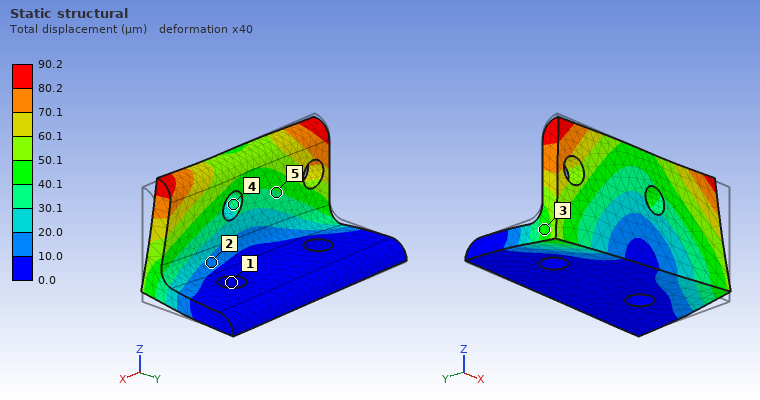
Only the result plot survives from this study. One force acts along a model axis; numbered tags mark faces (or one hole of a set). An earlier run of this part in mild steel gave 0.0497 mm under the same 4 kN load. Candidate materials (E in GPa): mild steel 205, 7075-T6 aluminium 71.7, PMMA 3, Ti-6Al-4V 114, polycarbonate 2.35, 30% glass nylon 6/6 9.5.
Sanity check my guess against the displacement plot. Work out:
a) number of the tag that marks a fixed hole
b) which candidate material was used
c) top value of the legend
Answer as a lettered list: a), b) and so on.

a) 1
b) Ti-6Al-4V
c) 90.2 µm
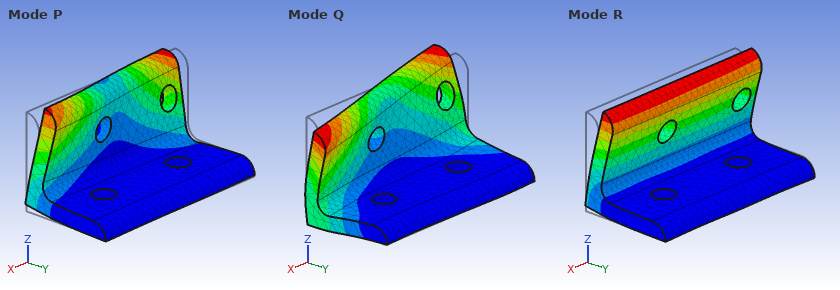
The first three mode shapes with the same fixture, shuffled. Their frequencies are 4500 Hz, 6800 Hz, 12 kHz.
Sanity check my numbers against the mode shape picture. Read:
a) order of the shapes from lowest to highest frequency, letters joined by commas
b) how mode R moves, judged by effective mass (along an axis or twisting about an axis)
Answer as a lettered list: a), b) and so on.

a) R, P, Q
b) along Y
